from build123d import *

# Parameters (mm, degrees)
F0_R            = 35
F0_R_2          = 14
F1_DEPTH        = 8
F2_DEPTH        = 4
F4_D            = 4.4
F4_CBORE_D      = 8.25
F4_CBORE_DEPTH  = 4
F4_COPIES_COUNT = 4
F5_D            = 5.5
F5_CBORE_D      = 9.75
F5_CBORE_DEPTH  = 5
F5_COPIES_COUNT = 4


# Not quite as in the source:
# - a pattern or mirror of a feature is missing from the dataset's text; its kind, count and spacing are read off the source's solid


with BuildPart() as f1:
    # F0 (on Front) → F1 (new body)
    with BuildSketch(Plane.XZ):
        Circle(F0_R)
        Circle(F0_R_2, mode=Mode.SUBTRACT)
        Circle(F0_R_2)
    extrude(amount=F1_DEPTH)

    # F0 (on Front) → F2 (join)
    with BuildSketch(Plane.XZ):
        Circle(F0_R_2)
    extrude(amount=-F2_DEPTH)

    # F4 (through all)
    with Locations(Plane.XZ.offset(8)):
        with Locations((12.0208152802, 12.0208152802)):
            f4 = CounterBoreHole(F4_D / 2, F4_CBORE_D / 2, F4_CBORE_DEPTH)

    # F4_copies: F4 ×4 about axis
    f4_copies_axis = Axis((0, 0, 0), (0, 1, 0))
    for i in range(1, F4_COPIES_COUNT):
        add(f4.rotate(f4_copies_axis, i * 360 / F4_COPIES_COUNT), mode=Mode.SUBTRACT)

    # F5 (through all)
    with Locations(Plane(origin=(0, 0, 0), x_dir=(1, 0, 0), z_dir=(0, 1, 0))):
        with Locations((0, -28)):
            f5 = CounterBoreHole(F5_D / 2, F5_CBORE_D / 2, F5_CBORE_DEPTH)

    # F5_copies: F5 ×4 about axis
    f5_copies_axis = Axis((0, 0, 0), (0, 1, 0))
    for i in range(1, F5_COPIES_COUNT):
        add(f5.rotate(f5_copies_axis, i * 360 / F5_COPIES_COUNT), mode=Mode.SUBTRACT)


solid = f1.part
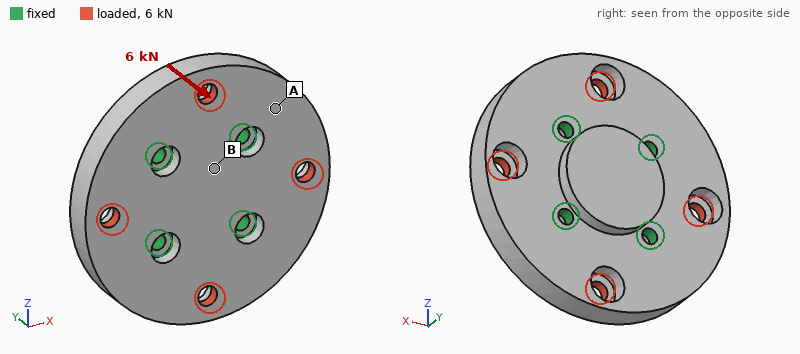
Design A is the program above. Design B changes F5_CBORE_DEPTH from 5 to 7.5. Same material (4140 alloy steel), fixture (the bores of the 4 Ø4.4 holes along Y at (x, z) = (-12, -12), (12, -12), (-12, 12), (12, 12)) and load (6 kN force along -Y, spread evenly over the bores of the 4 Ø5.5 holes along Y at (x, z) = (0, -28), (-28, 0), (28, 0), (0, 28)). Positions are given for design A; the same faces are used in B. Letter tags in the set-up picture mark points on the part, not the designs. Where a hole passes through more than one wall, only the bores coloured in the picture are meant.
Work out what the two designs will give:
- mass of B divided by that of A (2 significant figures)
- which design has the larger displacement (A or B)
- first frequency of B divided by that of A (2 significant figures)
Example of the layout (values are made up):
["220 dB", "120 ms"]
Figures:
["0.98", "B", "1.0"]
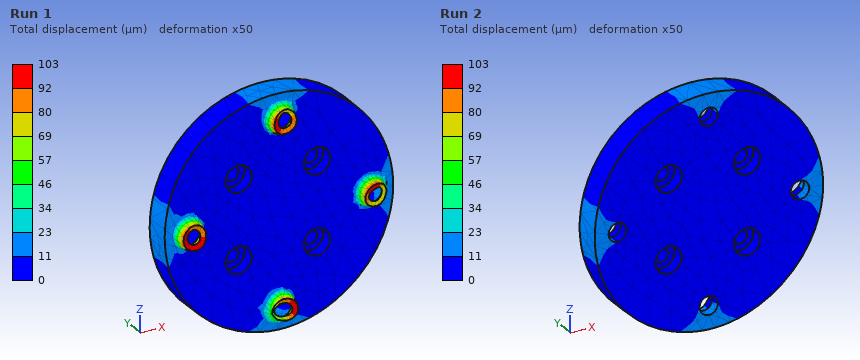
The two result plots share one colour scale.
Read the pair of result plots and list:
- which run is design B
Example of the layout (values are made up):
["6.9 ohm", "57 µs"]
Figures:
["Run 1"]
